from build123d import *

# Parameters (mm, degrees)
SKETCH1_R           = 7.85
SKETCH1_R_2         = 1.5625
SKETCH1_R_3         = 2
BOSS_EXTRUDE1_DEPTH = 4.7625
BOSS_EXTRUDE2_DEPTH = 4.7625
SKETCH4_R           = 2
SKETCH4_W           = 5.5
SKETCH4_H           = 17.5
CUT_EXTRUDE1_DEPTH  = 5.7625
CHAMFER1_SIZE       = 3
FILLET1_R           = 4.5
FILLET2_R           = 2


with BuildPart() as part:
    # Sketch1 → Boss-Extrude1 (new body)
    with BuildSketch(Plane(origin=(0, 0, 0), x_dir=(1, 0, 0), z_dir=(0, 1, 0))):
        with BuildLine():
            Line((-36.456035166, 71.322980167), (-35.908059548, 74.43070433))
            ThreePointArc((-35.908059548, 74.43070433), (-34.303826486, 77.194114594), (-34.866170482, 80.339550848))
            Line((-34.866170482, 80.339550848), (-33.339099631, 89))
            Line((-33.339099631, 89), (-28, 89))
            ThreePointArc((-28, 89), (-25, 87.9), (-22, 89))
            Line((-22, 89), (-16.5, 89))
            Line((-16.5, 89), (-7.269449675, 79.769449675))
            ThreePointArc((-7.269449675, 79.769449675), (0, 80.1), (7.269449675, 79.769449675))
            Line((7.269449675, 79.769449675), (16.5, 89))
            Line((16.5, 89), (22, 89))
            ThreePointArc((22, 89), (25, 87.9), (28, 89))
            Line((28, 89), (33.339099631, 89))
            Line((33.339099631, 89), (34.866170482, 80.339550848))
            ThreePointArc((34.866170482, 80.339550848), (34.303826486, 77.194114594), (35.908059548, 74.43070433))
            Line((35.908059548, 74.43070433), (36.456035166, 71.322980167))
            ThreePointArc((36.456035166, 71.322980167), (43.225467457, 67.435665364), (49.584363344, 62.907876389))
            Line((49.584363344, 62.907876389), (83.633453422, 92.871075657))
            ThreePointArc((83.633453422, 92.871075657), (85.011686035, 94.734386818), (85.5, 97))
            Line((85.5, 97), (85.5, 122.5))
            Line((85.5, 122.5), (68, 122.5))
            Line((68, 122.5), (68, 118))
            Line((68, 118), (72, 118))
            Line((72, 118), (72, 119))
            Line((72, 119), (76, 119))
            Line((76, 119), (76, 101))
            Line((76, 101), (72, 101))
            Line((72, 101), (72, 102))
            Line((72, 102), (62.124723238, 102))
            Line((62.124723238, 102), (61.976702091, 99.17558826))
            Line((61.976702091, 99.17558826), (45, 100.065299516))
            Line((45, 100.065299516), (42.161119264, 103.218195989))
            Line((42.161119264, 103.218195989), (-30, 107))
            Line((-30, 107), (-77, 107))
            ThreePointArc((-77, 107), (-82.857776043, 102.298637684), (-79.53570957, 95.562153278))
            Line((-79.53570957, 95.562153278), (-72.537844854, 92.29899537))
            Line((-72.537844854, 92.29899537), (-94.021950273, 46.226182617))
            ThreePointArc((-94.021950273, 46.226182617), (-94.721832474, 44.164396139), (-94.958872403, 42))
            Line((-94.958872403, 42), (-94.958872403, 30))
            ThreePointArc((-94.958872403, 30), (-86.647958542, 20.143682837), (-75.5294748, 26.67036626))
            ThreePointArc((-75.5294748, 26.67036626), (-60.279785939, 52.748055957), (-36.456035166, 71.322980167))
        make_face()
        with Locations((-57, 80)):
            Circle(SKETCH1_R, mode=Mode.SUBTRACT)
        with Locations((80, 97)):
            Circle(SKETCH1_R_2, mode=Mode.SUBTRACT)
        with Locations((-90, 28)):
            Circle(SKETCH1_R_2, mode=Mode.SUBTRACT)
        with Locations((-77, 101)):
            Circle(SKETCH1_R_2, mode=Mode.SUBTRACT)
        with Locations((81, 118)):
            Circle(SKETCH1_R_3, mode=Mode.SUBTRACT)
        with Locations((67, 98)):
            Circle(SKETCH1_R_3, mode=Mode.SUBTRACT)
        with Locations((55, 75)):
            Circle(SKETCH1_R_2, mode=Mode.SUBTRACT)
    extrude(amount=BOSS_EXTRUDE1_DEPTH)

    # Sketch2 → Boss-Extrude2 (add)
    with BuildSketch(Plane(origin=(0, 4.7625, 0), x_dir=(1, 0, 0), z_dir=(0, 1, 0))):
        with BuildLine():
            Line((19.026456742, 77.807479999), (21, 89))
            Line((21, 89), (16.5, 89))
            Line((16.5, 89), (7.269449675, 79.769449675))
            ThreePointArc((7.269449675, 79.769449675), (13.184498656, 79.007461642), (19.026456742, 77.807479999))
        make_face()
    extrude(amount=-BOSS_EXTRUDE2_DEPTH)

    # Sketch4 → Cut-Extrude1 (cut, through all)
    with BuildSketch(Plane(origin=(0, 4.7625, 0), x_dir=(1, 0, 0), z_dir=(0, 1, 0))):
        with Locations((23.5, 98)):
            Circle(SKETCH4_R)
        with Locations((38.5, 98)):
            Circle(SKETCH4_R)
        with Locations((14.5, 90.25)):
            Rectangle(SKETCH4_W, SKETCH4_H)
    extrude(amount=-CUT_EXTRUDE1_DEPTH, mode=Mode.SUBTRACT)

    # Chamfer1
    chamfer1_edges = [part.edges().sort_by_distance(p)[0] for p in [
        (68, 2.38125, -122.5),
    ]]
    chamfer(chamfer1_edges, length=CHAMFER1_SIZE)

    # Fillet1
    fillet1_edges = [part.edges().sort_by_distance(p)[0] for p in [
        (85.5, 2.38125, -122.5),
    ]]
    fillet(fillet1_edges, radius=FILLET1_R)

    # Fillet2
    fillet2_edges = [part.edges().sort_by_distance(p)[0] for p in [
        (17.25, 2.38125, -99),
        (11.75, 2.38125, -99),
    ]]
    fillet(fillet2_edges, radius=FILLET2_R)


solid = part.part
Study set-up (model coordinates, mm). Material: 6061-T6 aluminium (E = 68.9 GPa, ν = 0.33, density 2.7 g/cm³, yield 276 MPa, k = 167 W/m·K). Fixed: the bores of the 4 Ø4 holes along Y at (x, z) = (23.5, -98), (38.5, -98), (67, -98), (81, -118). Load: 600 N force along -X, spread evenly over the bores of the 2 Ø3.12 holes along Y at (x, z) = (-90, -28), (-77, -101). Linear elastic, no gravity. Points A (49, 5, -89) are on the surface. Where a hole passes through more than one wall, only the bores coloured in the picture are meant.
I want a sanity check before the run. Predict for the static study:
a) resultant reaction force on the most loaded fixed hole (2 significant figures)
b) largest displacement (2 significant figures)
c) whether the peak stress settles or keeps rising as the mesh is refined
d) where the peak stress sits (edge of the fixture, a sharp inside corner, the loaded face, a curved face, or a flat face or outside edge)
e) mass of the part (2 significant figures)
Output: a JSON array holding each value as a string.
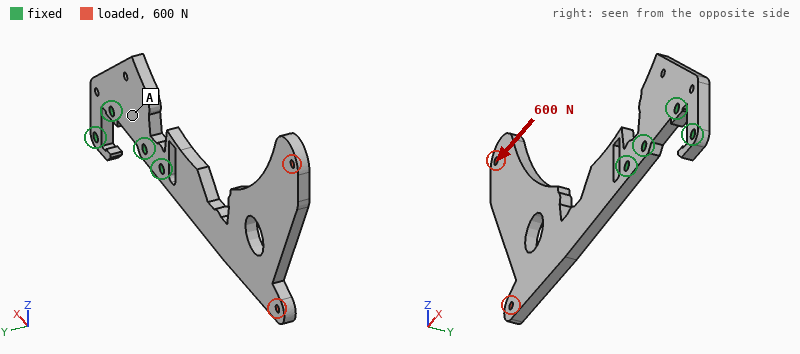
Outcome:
["810 N", "1.8 mm", "keeps rising", "a sharp inside corner", "72 g"]
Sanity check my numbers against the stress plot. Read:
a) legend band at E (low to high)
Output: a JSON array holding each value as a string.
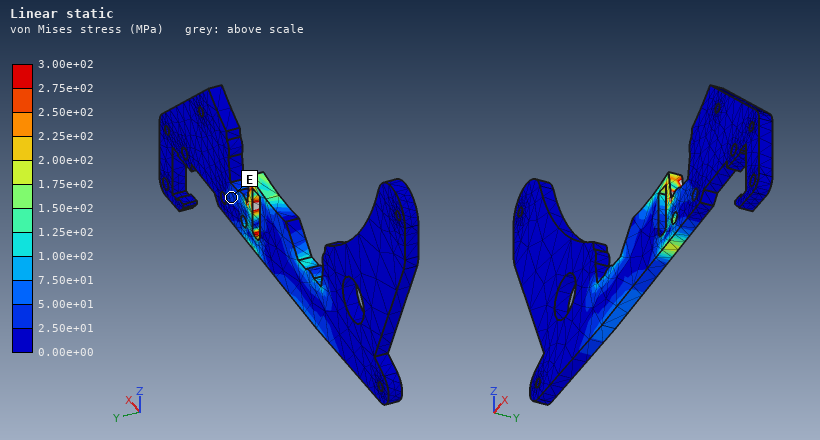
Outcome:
["2.50e+01 to 5.00e+01 MPa"]
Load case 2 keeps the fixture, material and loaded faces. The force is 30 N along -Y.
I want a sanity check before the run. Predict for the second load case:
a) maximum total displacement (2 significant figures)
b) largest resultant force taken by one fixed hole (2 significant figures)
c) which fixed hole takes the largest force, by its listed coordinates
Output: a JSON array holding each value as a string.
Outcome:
["2.2 mm", "74 N", "(23.5, -98)"]
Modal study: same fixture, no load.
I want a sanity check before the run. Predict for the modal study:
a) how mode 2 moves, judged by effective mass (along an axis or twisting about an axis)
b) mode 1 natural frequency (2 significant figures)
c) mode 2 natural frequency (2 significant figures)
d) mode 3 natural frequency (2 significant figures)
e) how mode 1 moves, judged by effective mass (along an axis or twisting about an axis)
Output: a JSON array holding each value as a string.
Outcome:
["along Z", "130 Hz", "370 Hz", "550 Hz", "along Y"]
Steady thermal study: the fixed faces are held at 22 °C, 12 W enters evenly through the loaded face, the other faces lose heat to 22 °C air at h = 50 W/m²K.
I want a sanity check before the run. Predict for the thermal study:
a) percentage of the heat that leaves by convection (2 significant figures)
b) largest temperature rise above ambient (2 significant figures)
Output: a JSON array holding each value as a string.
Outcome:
["77 %", "33 K"]
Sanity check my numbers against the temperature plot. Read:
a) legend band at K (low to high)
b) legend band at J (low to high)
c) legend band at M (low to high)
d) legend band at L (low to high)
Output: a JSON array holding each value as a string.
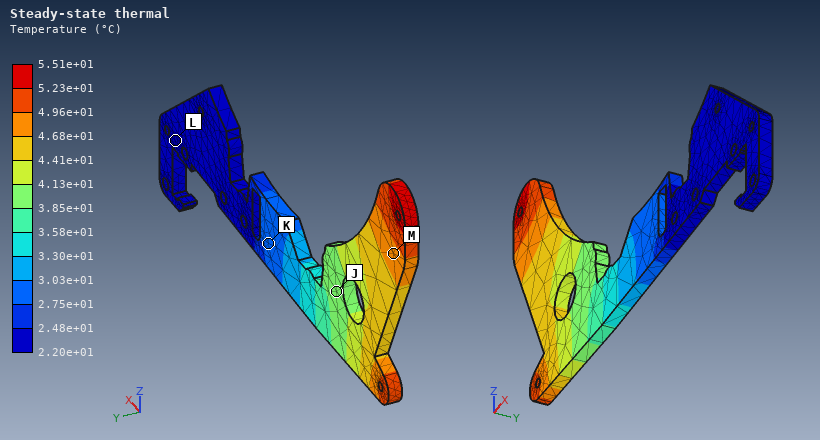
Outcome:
["2.75e+01 to 3.03e+01 °C", "3.85e+01 to 4.13e+01 °C", "4.68e+01 to 4.96e+01 °C", "2.20e+01 to 2.48e+01 °C"]
